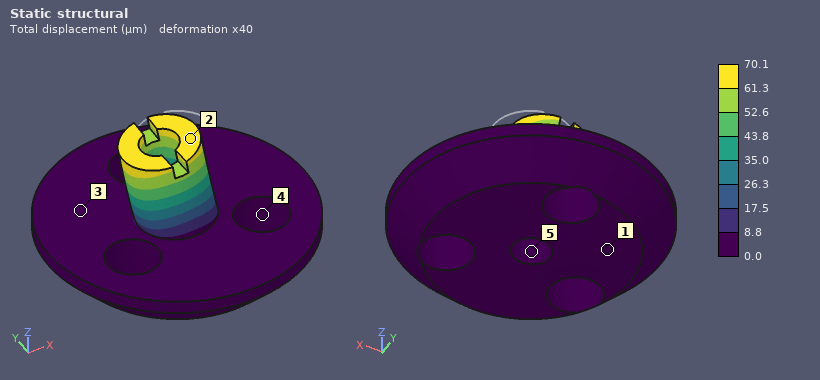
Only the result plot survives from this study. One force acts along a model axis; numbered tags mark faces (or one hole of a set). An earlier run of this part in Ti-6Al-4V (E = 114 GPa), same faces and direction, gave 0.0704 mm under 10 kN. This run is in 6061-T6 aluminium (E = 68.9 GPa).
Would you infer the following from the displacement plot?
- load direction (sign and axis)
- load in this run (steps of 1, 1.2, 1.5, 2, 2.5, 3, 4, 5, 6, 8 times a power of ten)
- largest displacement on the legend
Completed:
-X
6 kN
70.1 µm
